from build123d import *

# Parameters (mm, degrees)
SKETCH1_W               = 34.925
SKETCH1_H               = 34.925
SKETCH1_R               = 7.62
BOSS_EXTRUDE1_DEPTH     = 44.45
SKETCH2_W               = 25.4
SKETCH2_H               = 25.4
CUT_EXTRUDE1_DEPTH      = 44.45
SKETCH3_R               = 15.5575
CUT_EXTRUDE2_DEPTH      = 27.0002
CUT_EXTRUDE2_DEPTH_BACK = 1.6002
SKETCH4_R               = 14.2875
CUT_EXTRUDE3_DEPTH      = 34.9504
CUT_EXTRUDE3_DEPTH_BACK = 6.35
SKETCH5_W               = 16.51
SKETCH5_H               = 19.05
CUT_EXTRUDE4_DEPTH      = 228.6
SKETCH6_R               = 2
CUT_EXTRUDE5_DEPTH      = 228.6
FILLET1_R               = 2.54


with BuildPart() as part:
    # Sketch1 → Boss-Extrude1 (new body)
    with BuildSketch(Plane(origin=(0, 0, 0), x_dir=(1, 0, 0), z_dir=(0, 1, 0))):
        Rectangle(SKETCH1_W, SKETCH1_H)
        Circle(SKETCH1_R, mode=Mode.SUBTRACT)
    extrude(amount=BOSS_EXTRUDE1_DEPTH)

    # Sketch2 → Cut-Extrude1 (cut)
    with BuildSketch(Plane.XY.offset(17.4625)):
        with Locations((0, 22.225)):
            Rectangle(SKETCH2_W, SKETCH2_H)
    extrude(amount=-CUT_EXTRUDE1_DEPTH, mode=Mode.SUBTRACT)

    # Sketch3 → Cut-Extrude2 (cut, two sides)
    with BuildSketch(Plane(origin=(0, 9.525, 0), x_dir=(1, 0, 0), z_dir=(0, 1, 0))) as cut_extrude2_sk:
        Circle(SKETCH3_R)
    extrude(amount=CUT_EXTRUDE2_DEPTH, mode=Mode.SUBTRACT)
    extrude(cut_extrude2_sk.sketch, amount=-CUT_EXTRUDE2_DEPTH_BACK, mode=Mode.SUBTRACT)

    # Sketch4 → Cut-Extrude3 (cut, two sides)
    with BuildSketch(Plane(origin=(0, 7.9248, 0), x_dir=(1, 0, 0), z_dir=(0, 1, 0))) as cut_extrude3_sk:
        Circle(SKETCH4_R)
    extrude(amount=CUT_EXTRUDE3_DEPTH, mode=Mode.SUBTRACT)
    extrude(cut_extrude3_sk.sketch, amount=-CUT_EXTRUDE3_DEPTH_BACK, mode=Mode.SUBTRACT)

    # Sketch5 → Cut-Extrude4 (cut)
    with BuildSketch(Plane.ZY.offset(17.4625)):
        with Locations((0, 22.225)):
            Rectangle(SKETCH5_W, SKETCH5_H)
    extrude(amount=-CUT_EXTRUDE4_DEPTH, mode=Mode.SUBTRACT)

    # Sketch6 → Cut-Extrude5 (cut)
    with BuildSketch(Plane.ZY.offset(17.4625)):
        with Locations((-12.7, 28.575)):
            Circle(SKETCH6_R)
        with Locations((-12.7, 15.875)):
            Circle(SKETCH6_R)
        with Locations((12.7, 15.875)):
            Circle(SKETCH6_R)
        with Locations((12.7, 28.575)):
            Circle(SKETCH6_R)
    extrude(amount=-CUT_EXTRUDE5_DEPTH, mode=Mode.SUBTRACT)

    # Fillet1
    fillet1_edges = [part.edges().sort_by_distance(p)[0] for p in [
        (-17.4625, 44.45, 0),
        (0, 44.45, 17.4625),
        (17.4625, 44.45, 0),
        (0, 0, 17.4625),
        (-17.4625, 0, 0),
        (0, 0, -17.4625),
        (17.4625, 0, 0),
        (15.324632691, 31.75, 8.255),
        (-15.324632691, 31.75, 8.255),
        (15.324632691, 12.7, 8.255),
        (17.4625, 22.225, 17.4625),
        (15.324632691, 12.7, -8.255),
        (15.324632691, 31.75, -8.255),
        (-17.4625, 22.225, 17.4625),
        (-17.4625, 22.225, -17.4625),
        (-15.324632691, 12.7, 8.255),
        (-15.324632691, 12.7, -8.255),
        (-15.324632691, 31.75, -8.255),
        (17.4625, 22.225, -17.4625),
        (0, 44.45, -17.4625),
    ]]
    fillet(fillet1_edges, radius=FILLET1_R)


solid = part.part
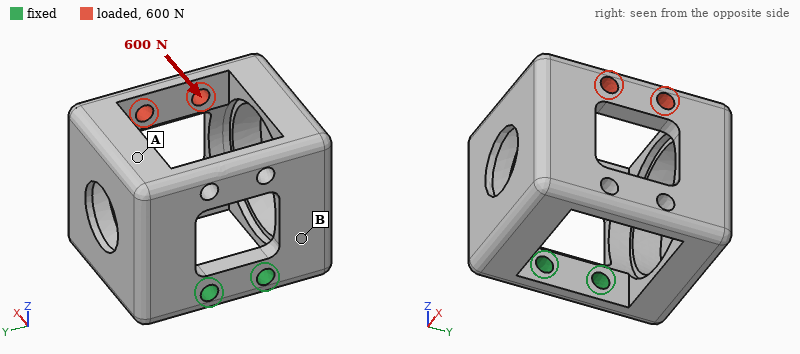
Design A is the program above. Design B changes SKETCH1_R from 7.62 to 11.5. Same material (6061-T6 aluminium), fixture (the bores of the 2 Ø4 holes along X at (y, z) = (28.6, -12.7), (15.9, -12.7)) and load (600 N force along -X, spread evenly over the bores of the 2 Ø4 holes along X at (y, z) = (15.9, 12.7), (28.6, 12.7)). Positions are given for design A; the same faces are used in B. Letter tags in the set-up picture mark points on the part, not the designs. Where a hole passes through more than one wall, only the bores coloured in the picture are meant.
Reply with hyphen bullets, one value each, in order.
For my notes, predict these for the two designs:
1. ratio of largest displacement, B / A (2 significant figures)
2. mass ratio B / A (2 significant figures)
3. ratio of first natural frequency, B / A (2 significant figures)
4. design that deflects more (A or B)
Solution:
- 1.2
- 0.95
- 0.95
- B
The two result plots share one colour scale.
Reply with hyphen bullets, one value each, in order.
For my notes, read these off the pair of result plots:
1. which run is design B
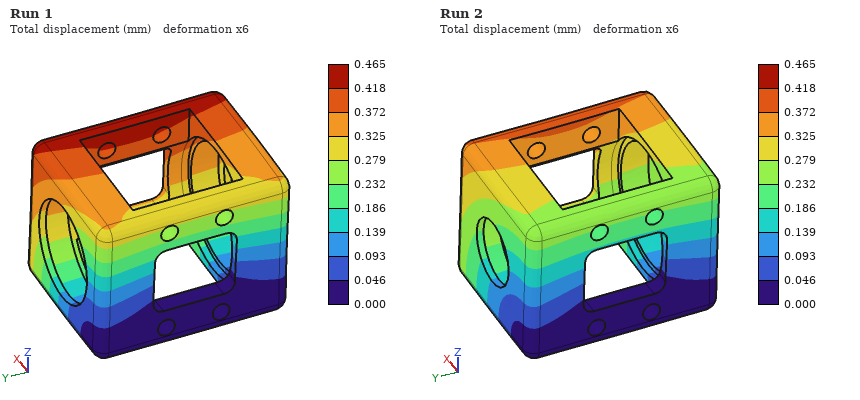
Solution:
- Run 1
